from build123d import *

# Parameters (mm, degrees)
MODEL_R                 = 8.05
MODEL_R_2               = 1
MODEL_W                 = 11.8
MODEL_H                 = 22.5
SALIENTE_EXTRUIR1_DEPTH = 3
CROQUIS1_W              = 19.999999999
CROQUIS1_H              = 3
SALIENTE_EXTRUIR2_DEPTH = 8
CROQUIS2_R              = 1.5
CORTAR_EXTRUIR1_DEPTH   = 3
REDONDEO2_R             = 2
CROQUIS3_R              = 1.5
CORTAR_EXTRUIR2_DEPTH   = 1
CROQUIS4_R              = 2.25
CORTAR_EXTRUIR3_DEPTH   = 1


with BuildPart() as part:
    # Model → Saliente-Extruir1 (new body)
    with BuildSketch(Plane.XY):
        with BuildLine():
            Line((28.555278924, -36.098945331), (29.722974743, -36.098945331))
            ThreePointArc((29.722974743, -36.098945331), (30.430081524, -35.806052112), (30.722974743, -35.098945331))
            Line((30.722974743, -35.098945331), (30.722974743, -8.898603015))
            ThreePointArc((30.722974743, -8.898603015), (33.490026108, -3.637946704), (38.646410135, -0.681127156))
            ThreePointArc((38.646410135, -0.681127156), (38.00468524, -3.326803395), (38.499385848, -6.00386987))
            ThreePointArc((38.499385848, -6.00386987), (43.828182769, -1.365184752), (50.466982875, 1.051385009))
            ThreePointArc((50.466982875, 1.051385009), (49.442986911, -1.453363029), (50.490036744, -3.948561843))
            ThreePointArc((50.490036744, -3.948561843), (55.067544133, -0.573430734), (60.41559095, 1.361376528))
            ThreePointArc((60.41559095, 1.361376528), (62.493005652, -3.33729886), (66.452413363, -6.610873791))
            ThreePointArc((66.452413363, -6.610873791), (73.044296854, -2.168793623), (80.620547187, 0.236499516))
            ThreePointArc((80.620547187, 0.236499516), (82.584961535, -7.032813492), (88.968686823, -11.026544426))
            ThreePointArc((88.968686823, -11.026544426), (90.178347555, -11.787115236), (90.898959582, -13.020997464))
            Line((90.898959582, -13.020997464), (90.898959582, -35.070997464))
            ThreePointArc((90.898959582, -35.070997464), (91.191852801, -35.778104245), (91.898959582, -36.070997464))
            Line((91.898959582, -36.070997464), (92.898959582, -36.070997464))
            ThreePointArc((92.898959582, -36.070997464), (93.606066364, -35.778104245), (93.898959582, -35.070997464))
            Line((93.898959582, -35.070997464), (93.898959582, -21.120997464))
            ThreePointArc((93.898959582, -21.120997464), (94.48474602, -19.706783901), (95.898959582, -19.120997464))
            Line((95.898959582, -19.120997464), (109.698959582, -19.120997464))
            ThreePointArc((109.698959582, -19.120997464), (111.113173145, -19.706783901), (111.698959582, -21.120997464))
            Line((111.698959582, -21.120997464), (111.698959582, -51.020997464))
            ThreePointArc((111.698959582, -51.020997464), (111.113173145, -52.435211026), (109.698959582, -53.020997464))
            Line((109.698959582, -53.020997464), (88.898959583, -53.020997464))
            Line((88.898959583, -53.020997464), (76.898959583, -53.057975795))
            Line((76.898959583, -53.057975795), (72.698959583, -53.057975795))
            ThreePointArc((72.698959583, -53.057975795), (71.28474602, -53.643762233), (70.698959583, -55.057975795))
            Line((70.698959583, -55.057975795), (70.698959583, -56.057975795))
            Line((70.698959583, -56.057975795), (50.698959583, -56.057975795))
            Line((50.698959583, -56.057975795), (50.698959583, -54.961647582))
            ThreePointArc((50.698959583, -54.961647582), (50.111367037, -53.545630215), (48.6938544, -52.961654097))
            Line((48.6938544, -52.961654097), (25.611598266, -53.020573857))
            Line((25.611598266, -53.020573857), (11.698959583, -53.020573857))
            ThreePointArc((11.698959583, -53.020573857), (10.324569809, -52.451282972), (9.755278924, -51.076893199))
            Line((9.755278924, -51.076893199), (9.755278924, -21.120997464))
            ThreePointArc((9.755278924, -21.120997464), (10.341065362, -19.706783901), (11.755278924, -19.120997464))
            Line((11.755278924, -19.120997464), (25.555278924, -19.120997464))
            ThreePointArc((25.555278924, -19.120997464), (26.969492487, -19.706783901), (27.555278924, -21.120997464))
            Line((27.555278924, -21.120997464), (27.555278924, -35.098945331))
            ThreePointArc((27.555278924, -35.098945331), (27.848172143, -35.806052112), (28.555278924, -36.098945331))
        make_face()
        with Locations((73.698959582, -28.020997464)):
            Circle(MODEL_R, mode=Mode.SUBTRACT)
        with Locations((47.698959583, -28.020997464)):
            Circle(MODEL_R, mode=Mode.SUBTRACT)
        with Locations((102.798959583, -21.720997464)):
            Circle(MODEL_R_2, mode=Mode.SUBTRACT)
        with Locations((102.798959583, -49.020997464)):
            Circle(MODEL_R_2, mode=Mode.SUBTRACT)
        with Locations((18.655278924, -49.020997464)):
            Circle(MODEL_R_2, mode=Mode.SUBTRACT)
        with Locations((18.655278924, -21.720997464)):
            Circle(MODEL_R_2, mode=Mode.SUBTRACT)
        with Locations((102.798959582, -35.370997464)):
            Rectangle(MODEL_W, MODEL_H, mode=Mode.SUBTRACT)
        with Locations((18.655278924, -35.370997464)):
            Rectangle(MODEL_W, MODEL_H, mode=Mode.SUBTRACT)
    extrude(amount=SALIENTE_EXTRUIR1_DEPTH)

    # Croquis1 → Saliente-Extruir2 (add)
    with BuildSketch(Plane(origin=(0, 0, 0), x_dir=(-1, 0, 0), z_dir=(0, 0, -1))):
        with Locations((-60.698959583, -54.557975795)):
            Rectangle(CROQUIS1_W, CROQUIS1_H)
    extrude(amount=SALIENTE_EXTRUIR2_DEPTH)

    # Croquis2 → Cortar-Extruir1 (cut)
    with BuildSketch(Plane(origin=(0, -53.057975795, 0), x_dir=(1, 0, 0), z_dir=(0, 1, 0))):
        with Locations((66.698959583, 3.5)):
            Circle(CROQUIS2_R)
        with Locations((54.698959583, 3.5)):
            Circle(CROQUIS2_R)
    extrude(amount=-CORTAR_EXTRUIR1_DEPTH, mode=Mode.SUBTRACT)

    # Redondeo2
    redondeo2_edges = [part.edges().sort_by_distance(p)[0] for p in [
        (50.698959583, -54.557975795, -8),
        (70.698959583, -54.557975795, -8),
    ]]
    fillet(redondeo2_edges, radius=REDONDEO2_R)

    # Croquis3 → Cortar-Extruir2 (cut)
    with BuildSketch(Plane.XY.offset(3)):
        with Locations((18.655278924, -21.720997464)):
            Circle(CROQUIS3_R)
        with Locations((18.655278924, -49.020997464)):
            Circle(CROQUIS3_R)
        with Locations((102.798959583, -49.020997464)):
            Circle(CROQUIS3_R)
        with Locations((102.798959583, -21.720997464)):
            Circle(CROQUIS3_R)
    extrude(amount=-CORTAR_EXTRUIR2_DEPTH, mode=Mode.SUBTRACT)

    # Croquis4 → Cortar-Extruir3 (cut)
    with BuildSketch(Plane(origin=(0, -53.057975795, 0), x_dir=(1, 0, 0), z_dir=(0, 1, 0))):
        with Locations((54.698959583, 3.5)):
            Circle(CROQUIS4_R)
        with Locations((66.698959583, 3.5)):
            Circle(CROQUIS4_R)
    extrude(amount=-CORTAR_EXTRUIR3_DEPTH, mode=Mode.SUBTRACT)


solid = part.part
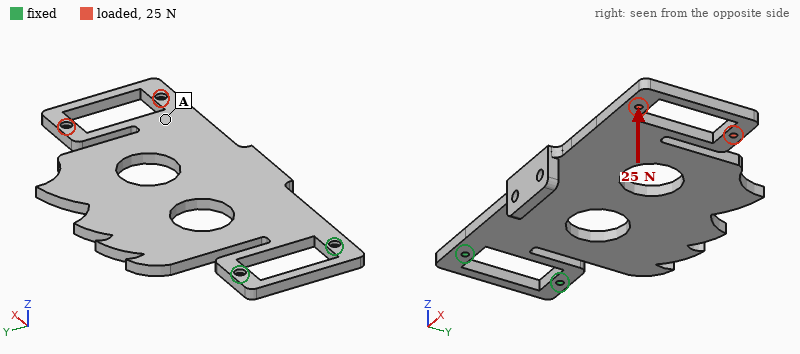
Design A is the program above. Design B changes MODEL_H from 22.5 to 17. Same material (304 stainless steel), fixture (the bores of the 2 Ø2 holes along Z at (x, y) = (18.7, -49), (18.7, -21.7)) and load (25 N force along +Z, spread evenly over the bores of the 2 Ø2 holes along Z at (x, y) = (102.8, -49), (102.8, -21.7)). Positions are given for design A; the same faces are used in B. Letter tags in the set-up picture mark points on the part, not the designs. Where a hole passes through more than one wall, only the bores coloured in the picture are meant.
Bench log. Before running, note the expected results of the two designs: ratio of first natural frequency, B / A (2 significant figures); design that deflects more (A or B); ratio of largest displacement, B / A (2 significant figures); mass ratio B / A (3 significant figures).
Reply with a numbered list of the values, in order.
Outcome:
1. 1.1
2. A
3. 0.85
4. 1.04
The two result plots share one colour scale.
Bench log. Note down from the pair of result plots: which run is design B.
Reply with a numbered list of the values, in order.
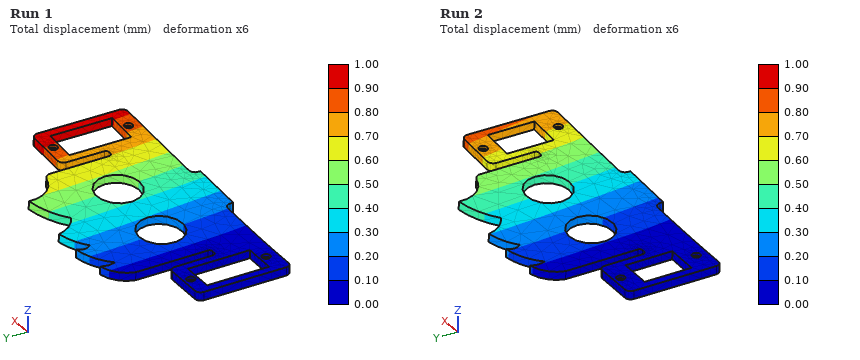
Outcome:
1. Run 2
